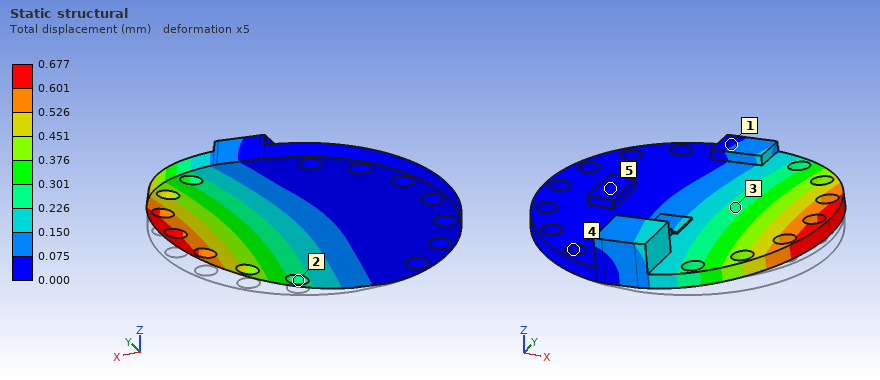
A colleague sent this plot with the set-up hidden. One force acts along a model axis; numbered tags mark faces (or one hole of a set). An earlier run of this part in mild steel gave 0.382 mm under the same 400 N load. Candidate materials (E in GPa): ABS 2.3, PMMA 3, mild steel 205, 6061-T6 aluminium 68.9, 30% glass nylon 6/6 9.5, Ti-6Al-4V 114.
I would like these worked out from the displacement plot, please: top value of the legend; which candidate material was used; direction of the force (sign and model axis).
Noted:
0.677 mm
Ti-6Al-4V
+Z
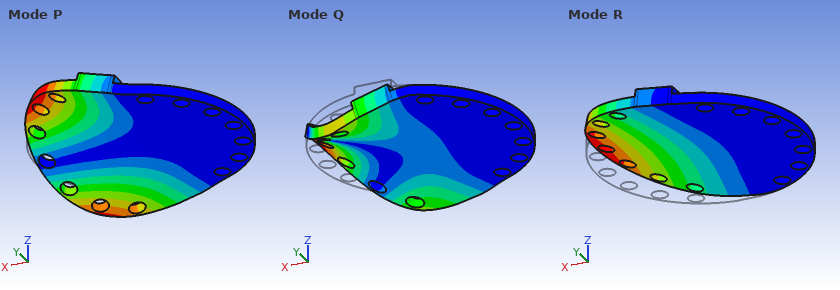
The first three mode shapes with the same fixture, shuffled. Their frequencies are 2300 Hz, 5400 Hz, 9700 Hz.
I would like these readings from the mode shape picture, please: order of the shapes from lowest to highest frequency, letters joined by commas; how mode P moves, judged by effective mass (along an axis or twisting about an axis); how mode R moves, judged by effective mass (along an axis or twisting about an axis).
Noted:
R, P, Q
twisting about X
along Z
